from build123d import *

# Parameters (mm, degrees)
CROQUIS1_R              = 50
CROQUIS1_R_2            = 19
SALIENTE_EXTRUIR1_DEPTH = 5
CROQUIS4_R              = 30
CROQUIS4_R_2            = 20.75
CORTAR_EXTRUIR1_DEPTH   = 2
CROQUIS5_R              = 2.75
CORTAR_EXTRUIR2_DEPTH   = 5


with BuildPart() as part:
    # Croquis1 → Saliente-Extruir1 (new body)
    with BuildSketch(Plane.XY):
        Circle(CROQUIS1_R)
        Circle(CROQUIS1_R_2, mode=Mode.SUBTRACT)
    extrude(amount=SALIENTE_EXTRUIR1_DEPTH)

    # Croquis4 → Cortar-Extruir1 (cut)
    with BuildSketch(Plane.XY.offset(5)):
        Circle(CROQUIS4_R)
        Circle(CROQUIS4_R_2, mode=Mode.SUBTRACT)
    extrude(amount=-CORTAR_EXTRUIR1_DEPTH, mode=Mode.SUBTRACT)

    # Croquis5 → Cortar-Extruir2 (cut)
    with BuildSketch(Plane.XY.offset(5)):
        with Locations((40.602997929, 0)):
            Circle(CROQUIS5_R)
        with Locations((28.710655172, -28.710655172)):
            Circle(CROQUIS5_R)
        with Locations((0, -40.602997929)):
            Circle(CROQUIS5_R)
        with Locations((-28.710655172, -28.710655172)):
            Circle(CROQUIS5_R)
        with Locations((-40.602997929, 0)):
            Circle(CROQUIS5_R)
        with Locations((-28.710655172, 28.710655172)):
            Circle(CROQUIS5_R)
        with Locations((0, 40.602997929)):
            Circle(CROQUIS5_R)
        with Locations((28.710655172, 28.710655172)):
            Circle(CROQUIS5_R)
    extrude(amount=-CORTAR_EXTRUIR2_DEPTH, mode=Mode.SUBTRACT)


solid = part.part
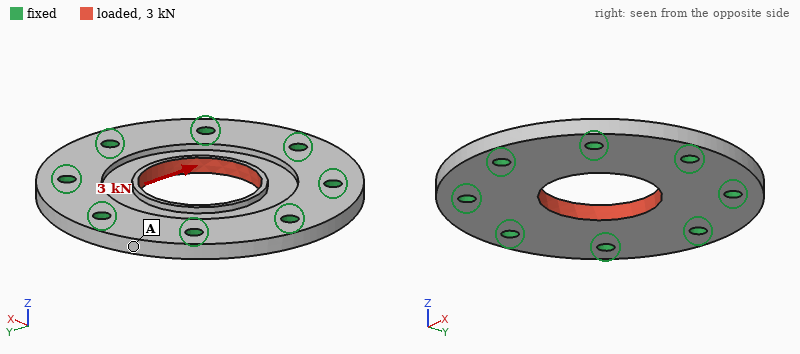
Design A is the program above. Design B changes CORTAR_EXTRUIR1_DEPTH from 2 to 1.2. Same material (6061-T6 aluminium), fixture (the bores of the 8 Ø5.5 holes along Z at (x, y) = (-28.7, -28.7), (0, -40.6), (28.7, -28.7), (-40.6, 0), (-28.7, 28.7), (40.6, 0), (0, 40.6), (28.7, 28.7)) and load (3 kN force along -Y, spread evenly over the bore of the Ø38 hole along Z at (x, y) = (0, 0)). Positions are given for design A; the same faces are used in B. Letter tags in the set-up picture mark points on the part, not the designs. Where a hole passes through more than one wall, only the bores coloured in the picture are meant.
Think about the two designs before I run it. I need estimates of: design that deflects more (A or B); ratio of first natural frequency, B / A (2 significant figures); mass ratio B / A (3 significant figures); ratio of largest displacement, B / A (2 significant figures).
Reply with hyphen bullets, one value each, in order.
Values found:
- A
- 0.99
- 1.04
- 0.54
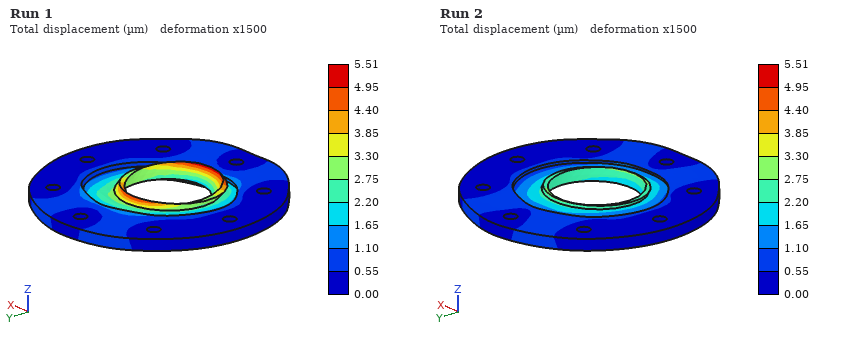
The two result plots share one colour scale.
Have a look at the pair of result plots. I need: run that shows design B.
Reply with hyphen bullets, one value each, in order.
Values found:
- Run 2
